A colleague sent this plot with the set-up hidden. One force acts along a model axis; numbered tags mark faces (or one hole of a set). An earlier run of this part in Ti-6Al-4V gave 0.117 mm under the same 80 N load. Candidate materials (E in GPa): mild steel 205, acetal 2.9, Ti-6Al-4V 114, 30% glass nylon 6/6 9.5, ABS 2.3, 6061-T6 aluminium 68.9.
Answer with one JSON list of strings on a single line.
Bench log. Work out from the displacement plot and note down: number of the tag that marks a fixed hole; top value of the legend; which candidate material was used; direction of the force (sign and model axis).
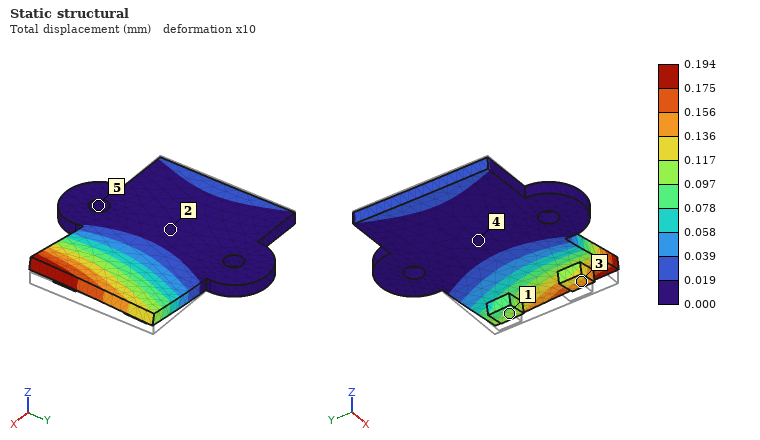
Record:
["5", "0.194 mm", "6061-T6 aluminium", "+Z"]
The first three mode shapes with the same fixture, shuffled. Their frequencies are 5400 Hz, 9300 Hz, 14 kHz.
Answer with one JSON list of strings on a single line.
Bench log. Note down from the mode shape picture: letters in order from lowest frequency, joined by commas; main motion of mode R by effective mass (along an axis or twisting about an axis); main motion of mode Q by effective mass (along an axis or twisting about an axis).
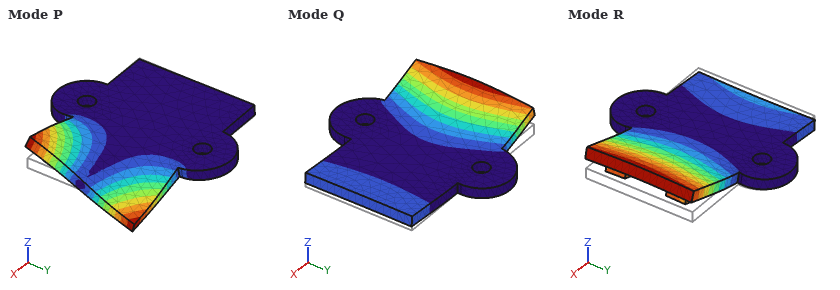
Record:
["R, Q, P", "along Z", "along Z"]
